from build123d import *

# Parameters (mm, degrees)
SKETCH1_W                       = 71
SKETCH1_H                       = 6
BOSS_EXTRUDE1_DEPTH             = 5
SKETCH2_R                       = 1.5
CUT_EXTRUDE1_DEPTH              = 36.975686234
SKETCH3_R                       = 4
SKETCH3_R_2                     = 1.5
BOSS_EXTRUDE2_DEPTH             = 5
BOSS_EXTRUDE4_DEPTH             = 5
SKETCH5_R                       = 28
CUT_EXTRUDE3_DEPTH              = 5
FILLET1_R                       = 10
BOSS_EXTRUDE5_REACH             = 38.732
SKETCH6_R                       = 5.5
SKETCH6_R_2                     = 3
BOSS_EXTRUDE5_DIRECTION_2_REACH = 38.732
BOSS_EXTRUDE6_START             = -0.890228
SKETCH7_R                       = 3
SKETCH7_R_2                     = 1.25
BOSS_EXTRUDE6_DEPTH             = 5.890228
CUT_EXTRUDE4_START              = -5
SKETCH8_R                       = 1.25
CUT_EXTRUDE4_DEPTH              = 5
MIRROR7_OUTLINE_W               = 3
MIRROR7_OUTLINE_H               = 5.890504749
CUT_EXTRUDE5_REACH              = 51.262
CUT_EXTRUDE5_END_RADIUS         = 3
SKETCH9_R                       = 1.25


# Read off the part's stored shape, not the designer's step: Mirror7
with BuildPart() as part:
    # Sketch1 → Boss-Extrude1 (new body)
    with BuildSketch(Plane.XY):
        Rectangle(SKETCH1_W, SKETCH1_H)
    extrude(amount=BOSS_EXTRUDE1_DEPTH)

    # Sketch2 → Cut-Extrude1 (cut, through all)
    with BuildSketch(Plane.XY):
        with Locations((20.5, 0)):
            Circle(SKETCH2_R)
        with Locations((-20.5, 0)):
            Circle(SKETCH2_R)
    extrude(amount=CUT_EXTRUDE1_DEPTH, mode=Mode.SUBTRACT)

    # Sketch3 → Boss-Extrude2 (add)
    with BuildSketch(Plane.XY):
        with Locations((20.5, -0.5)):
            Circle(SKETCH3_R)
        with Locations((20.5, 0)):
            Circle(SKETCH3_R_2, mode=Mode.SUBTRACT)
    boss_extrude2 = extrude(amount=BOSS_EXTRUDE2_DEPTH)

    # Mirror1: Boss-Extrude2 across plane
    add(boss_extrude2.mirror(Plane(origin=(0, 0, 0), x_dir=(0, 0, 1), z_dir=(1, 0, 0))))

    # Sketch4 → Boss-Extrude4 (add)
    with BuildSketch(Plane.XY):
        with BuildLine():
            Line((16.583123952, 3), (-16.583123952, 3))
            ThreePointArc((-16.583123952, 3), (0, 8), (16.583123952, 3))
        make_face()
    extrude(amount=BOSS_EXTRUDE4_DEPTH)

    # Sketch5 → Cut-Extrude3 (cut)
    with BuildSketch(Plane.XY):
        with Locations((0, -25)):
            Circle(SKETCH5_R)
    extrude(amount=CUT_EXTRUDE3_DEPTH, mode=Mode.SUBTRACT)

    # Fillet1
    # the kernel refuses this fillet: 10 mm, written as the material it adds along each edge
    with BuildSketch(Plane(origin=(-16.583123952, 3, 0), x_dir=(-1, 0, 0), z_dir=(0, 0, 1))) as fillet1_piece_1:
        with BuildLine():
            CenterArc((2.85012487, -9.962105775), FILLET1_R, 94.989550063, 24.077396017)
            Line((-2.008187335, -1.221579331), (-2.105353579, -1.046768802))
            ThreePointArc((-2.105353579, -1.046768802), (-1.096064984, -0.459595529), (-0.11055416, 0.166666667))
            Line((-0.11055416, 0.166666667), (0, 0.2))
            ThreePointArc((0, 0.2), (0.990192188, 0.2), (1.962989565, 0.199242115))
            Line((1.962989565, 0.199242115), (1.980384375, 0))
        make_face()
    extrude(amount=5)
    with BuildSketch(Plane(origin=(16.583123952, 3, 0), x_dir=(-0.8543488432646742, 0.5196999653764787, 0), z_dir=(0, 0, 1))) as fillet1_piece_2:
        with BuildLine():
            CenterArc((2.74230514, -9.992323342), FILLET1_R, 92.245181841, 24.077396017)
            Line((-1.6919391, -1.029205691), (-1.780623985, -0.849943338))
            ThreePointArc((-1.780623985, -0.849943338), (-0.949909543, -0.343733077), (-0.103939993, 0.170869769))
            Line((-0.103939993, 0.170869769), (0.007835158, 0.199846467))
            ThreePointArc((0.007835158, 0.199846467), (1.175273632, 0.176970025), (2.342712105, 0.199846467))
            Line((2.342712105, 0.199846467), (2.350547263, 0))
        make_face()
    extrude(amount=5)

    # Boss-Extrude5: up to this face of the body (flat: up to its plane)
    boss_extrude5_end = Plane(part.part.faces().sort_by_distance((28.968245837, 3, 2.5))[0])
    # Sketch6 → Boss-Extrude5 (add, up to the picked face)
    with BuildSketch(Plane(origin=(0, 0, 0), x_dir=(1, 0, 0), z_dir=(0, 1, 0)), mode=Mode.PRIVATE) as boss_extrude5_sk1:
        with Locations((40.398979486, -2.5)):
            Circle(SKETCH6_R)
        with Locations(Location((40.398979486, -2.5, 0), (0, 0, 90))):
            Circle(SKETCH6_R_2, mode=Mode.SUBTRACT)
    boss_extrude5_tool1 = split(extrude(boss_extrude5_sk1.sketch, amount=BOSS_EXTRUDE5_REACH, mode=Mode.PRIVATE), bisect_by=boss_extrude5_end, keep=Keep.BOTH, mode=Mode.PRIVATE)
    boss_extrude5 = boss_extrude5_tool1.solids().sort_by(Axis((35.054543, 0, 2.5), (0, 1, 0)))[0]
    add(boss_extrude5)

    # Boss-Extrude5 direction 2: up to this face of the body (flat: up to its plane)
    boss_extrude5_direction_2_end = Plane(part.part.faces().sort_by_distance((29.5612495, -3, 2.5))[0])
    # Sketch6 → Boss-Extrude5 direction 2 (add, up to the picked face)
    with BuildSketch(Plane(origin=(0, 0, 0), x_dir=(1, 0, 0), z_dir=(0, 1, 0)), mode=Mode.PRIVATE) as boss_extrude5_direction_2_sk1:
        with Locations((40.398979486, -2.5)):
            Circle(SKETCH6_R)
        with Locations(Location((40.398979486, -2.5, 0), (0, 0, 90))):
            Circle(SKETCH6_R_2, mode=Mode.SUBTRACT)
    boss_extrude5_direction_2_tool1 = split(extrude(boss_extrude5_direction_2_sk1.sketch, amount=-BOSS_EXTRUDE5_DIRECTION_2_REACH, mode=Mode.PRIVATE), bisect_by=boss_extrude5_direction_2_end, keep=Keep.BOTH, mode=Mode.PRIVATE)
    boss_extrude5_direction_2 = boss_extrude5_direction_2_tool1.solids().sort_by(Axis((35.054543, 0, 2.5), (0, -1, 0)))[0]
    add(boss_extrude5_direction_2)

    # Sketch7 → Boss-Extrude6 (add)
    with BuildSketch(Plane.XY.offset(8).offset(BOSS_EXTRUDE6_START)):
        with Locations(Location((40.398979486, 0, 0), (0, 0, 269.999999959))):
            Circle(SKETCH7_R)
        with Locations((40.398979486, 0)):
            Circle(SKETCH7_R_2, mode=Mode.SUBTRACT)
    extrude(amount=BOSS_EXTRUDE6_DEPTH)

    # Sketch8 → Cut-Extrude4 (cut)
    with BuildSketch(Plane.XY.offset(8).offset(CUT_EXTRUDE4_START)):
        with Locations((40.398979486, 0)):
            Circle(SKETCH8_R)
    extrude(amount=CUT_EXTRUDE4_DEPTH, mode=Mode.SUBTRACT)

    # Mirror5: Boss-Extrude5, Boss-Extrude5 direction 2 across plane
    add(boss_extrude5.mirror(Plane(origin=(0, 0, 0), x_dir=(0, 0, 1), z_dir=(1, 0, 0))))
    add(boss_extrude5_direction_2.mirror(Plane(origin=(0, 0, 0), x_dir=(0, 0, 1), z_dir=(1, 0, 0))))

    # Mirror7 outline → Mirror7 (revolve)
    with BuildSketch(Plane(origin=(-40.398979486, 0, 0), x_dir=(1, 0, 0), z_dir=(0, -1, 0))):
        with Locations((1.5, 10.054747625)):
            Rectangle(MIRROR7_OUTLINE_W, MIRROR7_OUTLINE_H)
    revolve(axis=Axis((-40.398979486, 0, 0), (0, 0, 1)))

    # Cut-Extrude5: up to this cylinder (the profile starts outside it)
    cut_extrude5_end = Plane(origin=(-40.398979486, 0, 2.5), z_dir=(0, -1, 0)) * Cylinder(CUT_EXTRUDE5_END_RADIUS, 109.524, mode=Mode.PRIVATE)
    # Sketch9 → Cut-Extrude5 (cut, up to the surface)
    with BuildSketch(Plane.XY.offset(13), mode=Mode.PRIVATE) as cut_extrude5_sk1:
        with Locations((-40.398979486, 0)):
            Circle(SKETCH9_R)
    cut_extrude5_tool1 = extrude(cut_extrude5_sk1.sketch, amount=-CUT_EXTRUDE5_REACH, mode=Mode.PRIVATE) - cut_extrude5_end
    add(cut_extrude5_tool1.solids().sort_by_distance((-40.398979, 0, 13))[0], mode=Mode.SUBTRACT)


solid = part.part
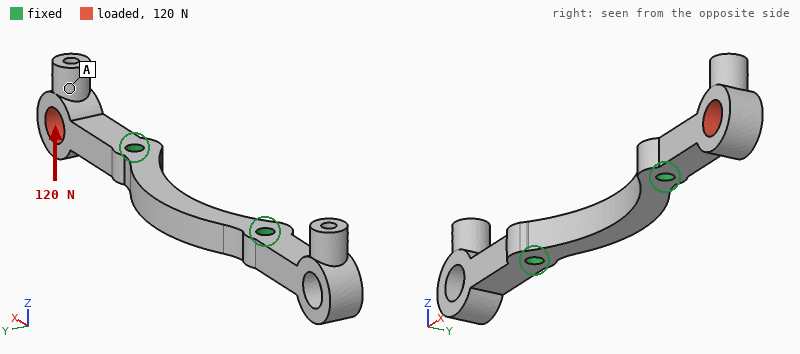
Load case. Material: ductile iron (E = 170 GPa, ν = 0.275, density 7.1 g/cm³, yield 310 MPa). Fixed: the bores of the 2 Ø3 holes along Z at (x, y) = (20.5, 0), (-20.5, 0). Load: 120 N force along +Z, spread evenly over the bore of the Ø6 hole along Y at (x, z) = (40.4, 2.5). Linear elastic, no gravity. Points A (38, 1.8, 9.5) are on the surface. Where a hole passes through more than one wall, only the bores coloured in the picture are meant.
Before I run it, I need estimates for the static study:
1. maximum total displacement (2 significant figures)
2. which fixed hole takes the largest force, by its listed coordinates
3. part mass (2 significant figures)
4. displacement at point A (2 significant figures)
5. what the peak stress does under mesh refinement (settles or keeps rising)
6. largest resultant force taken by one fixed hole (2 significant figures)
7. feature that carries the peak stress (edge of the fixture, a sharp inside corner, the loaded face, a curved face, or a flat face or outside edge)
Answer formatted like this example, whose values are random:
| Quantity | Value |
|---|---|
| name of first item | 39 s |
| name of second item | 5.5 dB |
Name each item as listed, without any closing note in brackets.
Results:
| Quantity | Value |
|---|---|
| maximum total displacement | 42 µm |
| which fixed hole takes the largest force, by its listed coordinates | (20.5, 0) |
| part mass | 21 g |
| displacement at point A | 27 µm |
| what the peak stress does under mesh refinement | keeps rising |
| largest resultant force taken by one fixed hole | 120 N |
| feature that carries the peak stress | edge of the fixture |
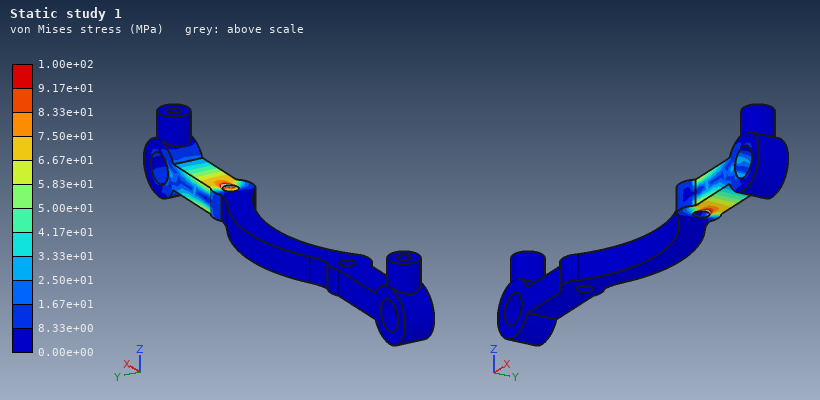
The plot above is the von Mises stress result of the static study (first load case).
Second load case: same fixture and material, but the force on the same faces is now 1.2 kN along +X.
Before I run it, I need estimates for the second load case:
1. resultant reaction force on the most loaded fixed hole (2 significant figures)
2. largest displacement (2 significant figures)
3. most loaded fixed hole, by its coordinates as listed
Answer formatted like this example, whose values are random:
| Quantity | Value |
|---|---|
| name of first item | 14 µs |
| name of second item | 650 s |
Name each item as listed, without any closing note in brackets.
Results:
| Quantity | Value |
|---|---|
| resultant reaction force on the most loaded fixed hole | 1.2 kN |
| largest displacement | 9.0 µm |
| most loaded fixed hole, by its coordinates as listed | (20.5, 0) |
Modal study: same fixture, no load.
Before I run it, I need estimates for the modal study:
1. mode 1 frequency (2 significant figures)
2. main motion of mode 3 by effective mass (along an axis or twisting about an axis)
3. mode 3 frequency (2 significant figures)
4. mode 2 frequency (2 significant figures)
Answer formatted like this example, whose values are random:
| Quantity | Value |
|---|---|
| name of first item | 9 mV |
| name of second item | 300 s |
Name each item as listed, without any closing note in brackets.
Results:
| Quantity | Value |
|---|---|
| mode 1 frequency | 4900 Hz |
| main motion of mode 3 by effective mass | along Y |
| mode 3 frequency | 5700 Hz |
| mode 2 frequency | 4900 Hz |
